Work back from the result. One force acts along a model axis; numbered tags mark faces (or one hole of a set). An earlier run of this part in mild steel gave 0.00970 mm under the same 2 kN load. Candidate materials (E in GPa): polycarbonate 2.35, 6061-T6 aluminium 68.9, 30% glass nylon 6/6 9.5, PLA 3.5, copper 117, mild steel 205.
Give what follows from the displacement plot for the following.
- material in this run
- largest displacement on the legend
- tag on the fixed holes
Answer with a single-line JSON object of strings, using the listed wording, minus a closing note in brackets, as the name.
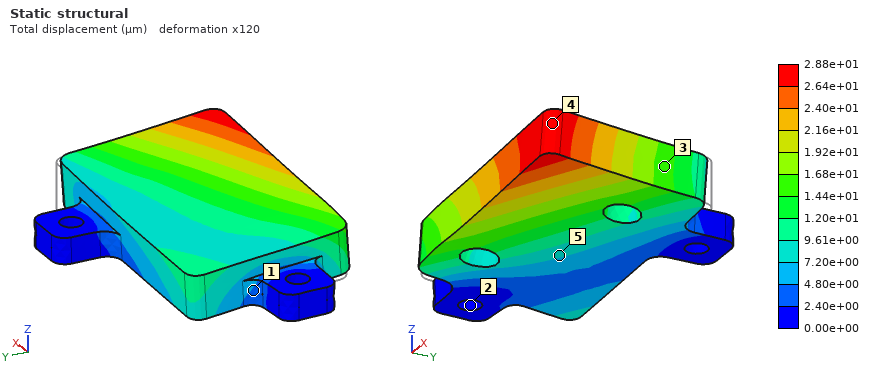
{"material in this run": "6061-T6 aluminium", "largest displacement on the legend": "2.88e+01 µm", "tag on the fixed holes": "2"}
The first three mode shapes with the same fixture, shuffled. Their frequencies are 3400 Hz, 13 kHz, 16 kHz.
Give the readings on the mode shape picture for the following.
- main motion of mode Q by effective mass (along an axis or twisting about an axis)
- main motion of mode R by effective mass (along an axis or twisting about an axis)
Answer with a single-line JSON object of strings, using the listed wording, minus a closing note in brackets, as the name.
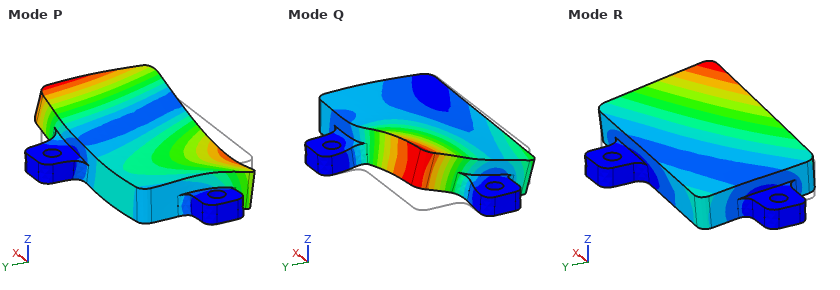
{"main motion of mode Q by effective mass": "along Z", "main motion of mode R by effective mass": "along Z"}
